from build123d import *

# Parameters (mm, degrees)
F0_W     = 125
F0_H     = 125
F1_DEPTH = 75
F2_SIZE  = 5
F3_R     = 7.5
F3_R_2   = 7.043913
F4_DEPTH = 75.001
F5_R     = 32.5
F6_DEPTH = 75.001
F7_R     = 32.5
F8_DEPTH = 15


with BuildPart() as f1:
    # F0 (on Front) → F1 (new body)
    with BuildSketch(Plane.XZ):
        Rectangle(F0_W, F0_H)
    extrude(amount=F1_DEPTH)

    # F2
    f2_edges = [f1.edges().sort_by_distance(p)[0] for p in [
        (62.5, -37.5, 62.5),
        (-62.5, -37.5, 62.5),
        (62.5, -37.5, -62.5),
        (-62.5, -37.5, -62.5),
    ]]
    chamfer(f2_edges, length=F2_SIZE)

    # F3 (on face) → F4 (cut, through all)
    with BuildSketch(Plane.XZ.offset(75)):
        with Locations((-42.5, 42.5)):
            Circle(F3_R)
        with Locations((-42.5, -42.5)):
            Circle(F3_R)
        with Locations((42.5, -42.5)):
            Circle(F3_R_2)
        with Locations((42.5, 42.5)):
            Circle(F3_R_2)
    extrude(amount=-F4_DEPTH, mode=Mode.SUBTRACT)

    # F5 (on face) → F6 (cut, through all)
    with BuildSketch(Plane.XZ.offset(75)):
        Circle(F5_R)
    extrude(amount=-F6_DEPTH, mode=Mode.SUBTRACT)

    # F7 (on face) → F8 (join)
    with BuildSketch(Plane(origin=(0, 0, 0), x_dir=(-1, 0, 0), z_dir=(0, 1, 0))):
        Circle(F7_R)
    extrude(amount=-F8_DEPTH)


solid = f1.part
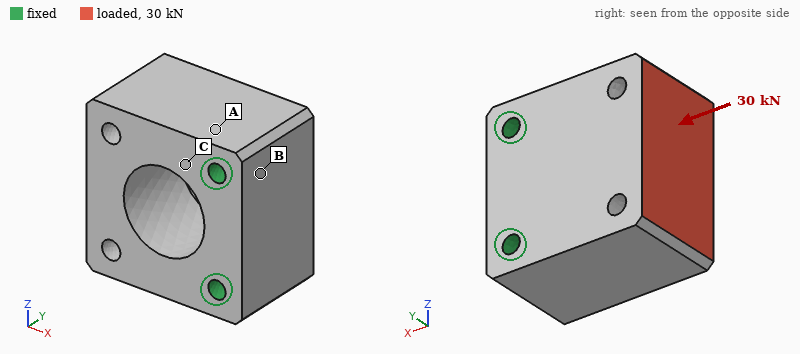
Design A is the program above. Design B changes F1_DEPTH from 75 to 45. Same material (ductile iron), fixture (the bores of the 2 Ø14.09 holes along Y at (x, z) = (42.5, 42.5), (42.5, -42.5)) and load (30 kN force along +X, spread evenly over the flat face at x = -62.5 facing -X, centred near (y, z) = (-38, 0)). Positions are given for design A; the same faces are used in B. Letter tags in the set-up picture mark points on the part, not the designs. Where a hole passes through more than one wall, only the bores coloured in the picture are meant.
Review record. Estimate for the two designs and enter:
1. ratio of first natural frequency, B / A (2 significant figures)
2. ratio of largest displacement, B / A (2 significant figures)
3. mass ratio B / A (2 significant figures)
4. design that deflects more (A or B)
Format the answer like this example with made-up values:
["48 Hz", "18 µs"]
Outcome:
["0.71", "1.7", "0.62", "B"]
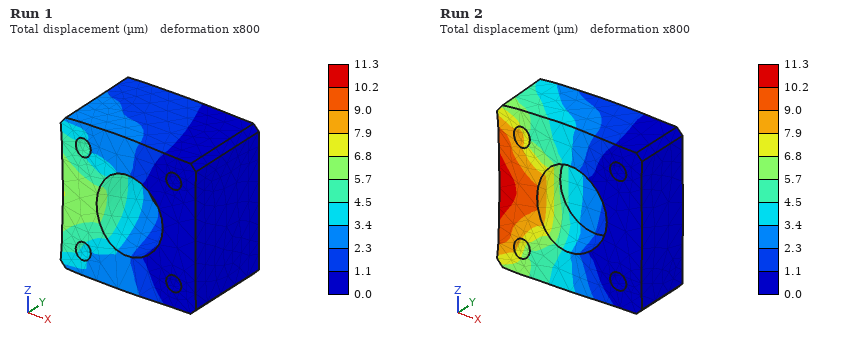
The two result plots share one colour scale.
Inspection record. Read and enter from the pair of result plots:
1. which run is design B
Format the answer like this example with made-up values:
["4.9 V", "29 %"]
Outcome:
["Run 2"]
